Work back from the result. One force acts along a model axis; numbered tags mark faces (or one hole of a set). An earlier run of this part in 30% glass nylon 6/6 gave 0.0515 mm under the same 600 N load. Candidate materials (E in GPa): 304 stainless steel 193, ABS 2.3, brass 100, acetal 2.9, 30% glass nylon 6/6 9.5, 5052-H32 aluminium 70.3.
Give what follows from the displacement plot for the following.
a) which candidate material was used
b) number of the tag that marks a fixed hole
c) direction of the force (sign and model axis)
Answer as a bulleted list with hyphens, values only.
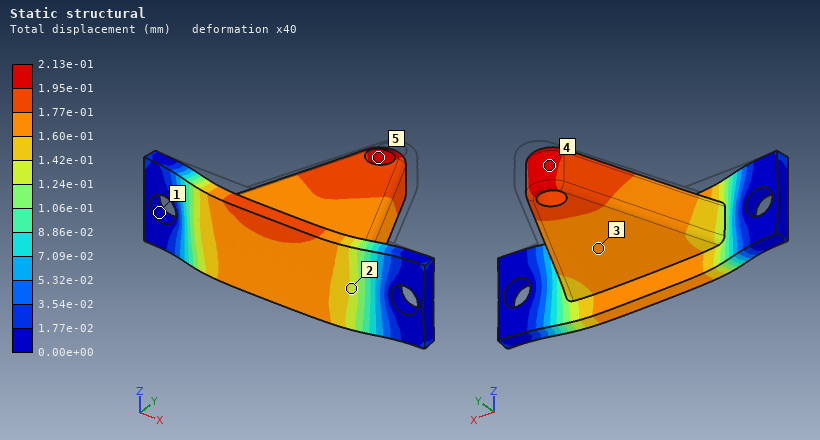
- ABS
- 1
- -Y
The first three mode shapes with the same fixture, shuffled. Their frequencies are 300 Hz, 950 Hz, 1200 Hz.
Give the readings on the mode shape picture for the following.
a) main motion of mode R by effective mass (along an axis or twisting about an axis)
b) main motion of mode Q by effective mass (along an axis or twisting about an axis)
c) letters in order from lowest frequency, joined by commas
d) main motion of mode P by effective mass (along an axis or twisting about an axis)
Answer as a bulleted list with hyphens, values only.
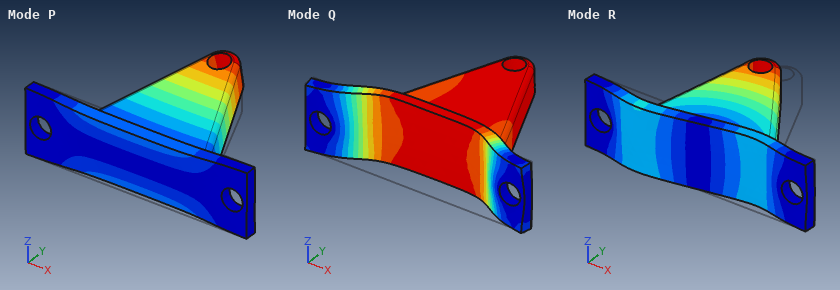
- along X
- along Y
- P, Q, R
- along Z
